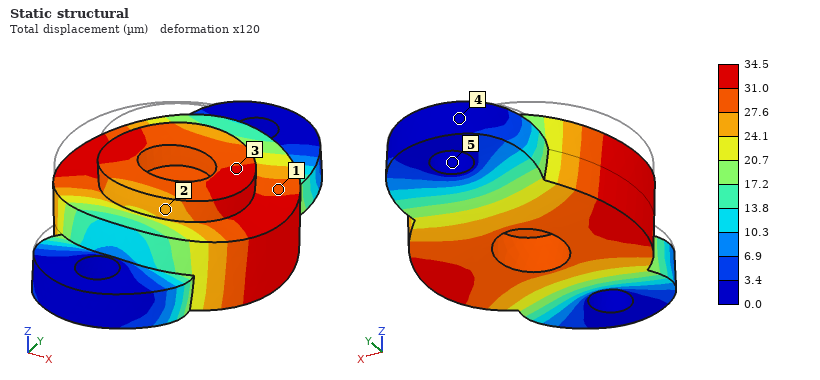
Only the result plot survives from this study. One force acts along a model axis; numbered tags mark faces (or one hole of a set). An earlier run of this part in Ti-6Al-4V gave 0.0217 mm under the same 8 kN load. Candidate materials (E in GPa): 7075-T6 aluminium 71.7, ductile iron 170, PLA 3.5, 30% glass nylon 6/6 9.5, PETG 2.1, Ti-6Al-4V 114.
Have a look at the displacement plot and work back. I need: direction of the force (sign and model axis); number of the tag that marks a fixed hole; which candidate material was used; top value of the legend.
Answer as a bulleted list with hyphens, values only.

- -Z
- 5
- 7075-T6 aluminium
- 34.5 µm
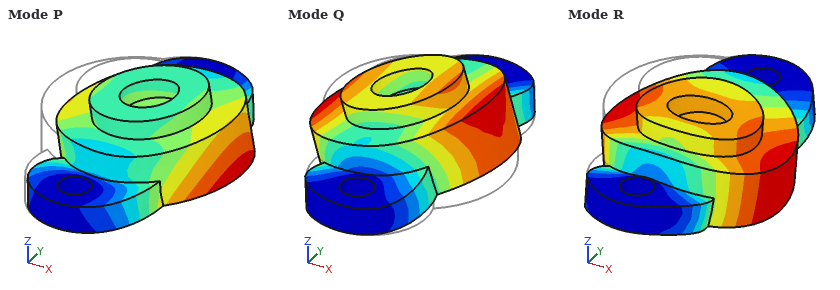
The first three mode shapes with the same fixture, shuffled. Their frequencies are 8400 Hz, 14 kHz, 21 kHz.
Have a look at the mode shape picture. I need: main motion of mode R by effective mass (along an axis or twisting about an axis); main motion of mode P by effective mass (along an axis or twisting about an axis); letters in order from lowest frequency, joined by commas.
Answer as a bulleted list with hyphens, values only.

- along Z
- along X
- Q, R, P
